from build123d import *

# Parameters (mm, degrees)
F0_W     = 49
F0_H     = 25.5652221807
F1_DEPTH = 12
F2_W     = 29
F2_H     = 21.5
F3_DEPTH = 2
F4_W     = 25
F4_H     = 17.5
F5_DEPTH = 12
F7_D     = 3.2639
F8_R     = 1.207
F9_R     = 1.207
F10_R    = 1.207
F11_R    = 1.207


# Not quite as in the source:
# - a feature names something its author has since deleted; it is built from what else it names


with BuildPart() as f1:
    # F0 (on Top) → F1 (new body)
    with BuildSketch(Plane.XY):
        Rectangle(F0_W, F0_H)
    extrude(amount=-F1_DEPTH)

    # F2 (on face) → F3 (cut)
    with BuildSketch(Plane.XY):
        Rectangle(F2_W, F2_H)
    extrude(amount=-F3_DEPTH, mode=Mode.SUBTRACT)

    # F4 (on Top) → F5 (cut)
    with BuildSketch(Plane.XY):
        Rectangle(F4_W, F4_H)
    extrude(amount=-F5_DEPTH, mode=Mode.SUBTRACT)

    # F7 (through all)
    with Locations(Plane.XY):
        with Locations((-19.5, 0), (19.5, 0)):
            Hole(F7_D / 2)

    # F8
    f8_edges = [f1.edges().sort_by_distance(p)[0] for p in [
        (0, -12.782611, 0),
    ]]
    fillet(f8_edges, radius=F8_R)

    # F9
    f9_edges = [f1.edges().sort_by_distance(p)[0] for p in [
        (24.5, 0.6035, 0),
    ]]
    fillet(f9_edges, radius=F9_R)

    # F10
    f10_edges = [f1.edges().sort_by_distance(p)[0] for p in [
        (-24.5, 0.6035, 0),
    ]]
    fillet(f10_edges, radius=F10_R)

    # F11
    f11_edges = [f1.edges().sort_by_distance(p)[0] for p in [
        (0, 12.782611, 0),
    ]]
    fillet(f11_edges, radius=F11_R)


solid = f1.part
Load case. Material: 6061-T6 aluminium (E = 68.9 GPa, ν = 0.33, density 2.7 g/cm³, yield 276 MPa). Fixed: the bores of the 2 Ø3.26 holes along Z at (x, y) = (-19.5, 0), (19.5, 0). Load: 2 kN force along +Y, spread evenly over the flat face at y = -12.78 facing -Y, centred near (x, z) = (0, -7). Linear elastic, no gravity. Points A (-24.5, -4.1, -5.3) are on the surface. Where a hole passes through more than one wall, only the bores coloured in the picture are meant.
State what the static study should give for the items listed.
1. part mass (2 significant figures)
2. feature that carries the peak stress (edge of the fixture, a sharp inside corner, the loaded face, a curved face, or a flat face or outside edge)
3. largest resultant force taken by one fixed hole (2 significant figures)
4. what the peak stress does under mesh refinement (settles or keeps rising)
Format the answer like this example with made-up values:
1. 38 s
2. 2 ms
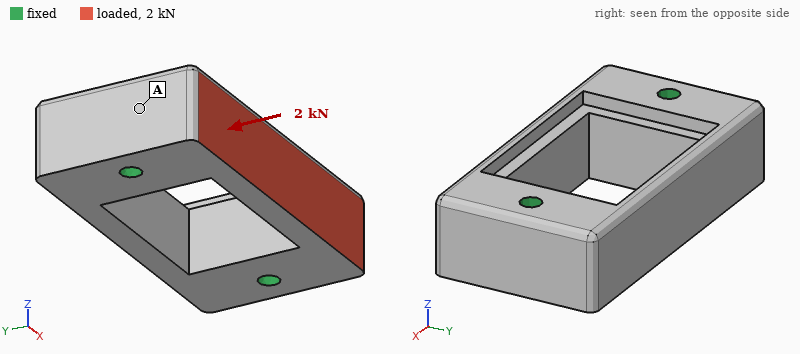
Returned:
1. 25 g
2. a sharp inside corner
3. 1.1 kN
4. keeps rising
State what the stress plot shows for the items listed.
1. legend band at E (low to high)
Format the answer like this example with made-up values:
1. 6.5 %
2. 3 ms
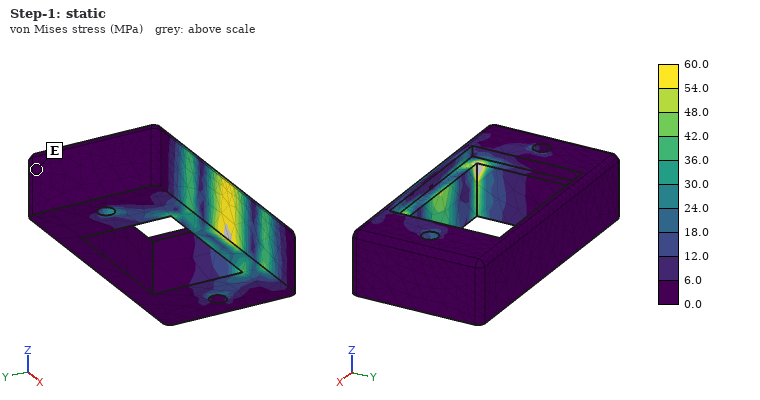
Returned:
1. 0.0 to 6.0 MPa
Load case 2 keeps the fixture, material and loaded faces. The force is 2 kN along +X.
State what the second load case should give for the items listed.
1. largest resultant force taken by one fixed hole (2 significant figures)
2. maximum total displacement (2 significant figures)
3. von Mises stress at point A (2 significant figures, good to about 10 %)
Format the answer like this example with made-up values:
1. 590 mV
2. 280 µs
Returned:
1. 1.0 kN
2. 16 µm
3. 22 MPa
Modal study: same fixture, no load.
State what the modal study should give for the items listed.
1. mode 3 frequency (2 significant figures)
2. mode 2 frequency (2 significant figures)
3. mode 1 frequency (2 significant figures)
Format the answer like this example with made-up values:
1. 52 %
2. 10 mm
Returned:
1. 21 kHz
2. 21 kHz
3. 18 kHz
